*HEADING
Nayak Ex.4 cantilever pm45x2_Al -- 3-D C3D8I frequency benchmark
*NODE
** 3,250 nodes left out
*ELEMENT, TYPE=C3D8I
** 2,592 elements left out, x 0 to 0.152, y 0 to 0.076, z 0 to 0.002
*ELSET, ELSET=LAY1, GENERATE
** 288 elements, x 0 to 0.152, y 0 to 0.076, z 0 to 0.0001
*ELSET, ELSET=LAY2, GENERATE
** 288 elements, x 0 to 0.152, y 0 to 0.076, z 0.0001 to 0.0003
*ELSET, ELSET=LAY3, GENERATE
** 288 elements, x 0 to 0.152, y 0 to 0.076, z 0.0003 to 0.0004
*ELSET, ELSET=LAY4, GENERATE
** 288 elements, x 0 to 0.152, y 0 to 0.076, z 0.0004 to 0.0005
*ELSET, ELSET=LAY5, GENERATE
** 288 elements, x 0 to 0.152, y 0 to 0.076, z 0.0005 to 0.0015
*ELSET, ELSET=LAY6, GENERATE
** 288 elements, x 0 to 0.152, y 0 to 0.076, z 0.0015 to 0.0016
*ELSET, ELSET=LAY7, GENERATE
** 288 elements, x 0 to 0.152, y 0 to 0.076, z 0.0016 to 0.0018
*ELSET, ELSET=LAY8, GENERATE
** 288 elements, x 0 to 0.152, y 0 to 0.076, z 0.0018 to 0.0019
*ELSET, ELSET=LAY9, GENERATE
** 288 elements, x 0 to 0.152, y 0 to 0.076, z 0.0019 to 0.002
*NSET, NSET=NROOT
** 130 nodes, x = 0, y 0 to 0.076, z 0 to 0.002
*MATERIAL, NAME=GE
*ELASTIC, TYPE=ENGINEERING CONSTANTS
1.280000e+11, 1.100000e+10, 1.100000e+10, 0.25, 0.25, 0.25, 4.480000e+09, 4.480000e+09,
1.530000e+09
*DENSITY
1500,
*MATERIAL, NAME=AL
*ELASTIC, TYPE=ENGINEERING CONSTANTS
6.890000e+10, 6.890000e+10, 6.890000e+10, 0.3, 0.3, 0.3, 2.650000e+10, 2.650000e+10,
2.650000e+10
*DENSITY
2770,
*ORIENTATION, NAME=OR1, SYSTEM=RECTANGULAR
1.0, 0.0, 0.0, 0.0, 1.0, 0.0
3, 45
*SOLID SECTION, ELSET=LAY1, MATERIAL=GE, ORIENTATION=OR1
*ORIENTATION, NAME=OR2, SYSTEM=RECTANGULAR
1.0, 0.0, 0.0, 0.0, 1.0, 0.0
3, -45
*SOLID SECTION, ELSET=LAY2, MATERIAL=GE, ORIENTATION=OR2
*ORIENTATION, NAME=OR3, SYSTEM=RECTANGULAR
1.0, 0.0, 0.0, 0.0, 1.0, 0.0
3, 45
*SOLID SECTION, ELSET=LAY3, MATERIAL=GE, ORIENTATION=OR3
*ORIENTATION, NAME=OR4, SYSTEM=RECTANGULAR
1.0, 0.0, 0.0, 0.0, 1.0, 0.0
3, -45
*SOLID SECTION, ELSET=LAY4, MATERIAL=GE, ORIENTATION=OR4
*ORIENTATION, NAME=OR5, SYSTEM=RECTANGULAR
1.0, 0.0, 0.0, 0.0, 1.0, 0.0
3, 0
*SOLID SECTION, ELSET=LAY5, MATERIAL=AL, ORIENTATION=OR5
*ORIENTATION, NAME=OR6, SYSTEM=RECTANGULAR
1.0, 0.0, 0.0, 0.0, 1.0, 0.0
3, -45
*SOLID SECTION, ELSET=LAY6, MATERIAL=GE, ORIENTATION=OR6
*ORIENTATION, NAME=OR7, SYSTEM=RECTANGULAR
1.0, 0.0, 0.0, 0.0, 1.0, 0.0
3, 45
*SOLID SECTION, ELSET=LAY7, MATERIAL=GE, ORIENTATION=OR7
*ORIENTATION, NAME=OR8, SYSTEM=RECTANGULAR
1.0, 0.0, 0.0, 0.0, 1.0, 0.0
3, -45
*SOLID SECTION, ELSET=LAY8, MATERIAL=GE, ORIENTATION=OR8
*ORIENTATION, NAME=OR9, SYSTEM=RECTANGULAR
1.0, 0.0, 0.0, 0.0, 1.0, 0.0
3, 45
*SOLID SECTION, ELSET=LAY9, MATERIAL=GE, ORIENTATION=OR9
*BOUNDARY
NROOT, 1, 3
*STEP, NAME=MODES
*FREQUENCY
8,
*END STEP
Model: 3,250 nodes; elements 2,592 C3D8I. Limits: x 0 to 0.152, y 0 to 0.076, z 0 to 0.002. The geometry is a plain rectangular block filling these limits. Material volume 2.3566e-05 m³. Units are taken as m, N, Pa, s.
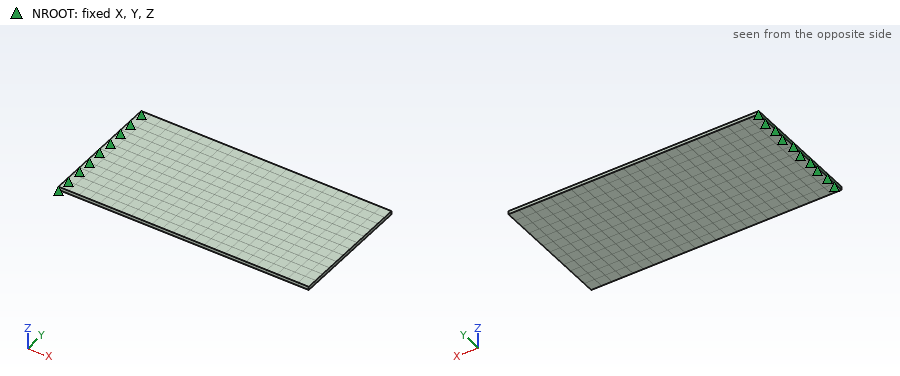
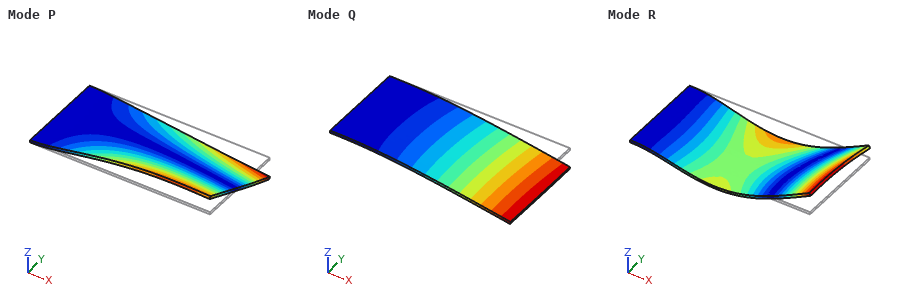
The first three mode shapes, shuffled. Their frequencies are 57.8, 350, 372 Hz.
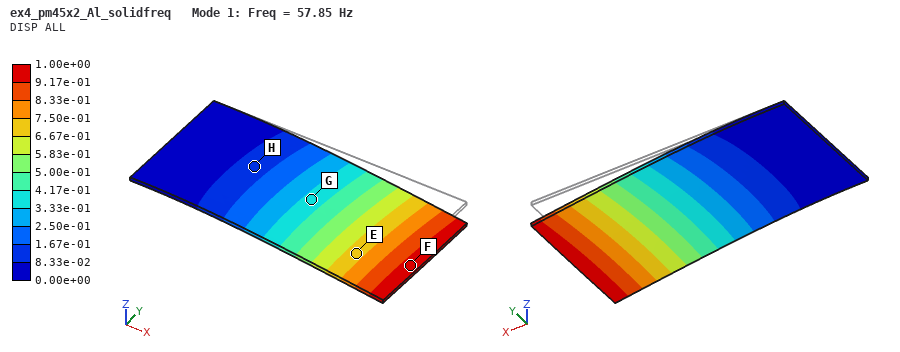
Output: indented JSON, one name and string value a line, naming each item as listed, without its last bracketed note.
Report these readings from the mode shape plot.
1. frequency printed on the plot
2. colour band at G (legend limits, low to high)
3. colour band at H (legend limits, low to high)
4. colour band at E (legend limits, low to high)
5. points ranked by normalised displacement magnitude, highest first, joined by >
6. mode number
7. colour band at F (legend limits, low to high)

{
  "frequency printed on the plot": "57.85 Hz",
  "colour band at G": "3.33e-01 to 4.17e-01",
  "colour band at H": "8.33e-02 to 1.67e-01",
  "colour band at E": "6.67e-01 to 7.50e-01",
  "points ranked by normalised displacement magnitude, highest first, joined by >": "F > E > G > H",
  "mode number": "1",
  "colour band at F": "9.17e-01 to 1.00e+00"
}
